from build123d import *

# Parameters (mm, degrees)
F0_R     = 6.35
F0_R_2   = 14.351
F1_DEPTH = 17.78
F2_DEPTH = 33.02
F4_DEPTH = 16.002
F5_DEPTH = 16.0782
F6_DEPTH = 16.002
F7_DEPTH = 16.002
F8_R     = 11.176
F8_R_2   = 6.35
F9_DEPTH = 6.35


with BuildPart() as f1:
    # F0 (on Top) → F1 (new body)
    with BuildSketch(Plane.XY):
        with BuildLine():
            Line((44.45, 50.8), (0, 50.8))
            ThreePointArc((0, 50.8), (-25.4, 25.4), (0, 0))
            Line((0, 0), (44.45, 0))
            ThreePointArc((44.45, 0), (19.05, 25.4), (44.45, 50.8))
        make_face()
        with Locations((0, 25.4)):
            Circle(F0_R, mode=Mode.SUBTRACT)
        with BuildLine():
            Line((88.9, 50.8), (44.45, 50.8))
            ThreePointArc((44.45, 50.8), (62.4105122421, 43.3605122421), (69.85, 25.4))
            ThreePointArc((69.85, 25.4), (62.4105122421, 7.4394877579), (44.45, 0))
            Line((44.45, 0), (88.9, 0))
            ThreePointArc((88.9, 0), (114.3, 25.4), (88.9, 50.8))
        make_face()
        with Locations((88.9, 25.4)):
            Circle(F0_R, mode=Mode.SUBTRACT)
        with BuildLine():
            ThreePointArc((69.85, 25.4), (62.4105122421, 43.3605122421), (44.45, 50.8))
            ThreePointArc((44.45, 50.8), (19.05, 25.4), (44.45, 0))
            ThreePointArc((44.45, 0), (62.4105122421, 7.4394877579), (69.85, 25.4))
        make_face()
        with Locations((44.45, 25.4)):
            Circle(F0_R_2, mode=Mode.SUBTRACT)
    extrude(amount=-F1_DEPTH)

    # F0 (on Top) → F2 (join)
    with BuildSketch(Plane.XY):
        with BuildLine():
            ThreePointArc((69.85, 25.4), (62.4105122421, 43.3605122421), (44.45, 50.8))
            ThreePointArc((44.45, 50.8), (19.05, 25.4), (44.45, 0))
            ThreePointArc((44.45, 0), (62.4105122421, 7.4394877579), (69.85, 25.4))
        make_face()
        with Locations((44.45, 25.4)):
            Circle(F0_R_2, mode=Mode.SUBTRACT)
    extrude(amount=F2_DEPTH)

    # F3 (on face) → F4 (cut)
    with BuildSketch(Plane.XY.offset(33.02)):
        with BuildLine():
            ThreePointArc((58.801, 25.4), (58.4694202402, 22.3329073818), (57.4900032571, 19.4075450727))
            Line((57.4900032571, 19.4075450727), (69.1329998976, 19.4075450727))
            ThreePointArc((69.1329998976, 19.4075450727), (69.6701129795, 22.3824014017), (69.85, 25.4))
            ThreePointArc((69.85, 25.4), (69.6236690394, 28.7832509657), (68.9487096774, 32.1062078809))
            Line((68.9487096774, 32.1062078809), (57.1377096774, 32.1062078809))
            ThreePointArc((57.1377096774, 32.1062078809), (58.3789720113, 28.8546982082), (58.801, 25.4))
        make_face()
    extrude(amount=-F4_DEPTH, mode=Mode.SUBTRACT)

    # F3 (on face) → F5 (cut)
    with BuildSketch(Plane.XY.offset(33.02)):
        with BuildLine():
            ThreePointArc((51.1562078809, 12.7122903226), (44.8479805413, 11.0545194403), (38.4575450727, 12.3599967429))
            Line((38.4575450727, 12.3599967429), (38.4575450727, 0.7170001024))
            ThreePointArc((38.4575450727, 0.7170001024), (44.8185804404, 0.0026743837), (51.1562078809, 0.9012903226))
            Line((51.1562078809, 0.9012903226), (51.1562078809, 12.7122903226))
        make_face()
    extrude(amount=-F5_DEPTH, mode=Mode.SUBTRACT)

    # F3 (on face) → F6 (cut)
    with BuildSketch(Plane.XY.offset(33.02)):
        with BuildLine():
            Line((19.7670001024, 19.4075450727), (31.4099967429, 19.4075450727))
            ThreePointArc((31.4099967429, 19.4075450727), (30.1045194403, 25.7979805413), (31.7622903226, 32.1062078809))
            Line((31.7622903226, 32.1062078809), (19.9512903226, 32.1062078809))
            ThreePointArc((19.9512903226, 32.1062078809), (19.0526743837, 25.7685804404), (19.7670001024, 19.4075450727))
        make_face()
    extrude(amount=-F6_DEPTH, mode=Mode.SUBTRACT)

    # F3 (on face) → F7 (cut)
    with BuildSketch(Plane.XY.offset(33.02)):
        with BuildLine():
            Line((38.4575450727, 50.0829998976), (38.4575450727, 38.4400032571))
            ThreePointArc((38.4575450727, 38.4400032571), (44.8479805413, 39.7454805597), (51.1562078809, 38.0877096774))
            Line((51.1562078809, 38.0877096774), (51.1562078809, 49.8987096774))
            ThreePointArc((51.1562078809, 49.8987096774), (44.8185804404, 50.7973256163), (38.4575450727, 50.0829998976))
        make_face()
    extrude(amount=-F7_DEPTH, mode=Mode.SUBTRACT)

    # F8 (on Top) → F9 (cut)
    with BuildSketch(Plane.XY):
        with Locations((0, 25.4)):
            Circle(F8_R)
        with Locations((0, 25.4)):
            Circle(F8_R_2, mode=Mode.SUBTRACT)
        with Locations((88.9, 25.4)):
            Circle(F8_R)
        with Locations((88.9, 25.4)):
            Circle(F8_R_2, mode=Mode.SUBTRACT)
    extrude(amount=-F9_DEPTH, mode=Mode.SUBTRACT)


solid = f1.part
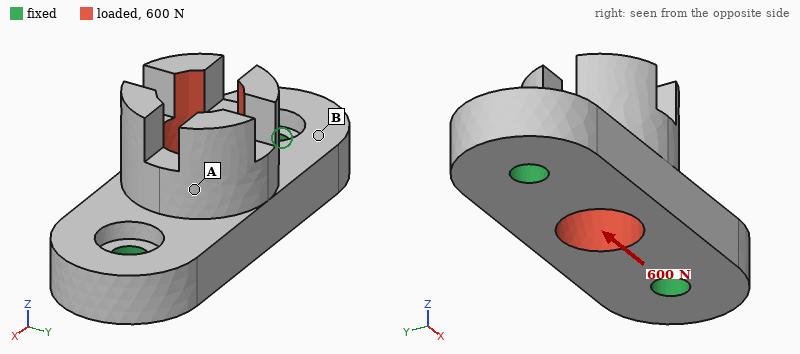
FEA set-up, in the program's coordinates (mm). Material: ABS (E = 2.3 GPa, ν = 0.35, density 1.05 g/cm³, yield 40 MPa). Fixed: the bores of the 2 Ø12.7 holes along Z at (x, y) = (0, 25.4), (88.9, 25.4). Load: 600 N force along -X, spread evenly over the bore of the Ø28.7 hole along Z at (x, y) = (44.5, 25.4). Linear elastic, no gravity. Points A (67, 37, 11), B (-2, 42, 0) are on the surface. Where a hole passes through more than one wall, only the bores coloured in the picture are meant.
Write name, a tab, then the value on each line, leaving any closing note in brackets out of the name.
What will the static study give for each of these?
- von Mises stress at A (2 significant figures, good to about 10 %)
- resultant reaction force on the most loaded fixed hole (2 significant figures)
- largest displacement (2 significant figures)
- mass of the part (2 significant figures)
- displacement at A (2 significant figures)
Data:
von Mises stress at A	0.54 MPa
resultant reaction force on the most loaded fixed hole	320 N
largest displacement	41 µm
mass of the part	140 g
displacement at A	17 µm
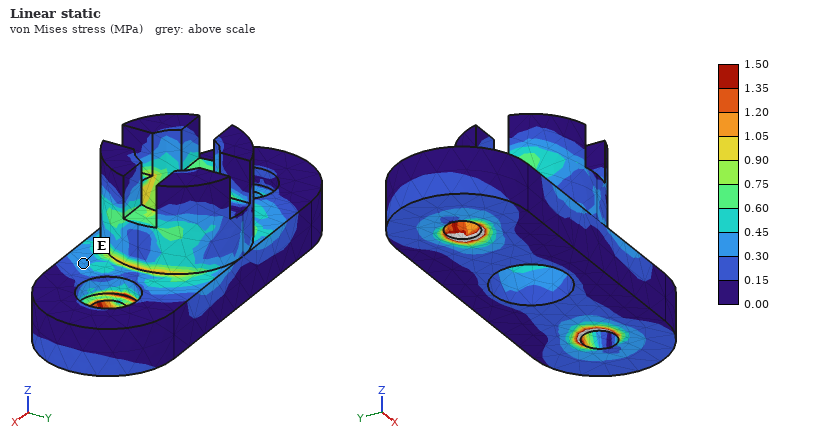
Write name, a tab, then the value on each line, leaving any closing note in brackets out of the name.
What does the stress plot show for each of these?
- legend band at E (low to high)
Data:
legend band at E	0.30 to 0.45 MPa
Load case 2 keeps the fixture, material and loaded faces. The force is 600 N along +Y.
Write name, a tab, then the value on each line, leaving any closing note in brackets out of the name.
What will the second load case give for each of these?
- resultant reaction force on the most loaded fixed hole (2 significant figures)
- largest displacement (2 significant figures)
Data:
resultant reaction force on the most loaded fixed hole	300 N
largest displacement	0.17 mm
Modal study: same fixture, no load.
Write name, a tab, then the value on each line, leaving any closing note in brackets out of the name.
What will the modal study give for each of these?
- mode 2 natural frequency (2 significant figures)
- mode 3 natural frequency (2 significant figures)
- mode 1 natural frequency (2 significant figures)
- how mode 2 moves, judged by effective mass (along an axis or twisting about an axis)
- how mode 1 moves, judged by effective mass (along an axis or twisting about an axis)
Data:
mode 2 natural frequency	2100 Hz
mode 3 natural frequency	2800 Hz
mode 1 natural frequency	1200 Hz
how mode 2 moves, judged by effective mass	along Z
how mode 1 moves, judged by effective mass	along Y
